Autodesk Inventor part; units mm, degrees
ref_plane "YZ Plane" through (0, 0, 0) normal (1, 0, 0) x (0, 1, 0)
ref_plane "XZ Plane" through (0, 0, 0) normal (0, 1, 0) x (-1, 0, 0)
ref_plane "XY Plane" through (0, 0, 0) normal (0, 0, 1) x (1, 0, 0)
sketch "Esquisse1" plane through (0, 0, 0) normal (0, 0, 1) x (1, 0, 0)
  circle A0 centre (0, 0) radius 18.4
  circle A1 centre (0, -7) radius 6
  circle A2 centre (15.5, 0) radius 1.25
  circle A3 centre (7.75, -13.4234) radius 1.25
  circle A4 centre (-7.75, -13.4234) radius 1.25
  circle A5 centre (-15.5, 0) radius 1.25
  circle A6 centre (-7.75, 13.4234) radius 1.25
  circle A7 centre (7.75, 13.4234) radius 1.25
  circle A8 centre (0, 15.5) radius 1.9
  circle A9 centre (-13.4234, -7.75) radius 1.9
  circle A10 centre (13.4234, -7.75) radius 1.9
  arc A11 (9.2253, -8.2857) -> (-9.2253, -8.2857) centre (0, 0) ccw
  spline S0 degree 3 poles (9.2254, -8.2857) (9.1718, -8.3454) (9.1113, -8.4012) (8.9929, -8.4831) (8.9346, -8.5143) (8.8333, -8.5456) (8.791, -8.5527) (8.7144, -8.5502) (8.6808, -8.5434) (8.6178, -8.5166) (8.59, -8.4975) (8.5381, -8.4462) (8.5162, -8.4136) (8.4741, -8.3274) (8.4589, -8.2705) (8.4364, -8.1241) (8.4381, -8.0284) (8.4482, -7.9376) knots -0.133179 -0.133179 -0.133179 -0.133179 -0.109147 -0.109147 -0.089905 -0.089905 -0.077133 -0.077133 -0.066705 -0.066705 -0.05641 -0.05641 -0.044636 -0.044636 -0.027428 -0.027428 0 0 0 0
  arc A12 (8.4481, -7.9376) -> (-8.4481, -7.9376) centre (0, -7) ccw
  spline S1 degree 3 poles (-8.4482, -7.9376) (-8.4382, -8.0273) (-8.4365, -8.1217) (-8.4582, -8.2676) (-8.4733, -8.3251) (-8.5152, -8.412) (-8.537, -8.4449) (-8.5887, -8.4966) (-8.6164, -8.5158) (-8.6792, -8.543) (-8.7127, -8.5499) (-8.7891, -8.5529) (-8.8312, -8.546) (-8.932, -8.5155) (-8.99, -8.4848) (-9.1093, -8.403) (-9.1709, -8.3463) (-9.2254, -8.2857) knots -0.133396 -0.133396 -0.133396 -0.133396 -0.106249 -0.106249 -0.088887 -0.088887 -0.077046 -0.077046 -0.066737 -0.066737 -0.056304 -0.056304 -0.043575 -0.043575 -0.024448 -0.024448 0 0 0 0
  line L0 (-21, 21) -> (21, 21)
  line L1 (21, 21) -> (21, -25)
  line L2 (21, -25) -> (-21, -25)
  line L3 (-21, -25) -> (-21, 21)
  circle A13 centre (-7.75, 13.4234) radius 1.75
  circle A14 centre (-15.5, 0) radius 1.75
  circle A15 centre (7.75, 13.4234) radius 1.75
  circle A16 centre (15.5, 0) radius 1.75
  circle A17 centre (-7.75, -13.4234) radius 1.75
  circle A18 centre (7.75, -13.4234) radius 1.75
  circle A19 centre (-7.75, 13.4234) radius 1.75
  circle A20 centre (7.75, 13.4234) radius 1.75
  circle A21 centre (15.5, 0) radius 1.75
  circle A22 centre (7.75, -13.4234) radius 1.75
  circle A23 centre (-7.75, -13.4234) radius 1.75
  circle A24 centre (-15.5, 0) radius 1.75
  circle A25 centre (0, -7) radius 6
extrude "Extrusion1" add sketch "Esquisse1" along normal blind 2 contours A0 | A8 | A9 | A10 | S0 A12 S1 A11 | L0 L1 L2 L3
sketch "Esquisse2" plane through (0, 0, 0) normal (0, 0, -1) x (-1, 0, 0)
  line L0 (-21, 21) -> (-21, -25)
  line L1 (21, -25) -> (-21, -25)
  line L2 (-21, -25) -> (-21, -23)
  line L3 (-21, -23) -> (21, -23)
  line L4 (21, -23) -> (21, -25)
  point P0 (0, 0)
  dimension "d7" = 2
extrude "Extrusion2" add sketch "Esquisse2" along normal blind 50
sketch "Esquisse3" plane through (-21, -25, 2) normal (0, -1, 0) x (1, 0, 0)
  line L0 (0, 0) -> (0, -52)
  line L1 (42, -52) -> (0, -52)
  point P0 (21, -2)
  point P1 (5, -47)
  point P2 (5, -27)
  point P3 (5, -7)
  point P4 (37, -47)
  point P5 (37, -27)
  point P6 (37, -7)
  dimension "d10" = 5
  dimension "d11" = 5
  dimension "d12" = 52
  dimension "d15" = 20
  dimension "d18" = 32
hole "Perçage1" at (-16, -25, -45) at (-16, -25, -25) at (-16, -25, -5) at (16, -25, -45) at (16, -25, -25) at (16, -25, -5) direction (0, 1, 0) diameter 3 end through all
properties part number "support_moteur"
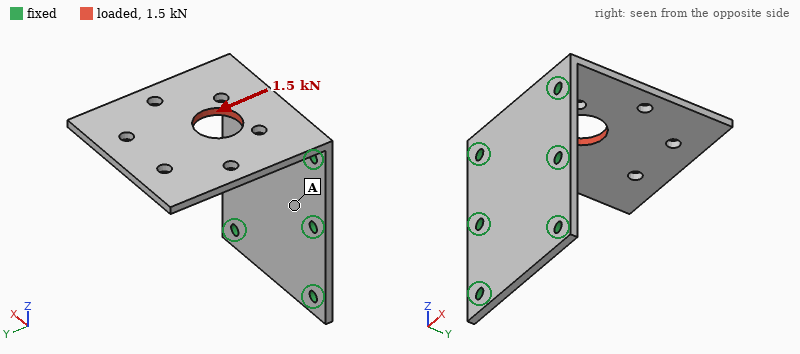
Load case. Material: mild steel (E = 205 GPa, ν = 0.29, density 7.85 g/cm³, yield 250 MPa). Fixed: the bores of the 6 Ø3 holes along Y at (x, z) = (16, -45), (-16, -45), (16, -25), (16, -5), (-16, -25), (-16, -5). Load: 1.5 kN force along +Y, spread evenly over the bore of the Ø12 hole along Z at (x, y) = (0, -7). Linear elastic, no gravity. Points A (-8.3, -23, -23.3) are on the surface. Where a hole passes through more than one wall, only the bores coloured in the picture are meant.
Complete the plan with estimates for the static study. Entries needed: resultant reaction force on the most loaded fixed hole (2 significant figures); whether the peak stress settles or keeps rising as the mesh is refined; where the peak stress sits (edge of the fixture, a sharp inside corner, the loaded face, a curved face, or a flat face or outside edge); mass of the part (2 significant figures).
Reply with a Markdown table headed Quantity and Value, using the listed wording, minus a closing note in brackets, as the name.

| Quantity | Value |
|---|---|
| resultant reaction force on the most loaded fixed hole | 810 N |
| whether the peak stress settles or keeps rising as the mesh is refined | keeps rising |
| where the peak stress sits | edge of the fixture |
| mass of the part | 60 g |
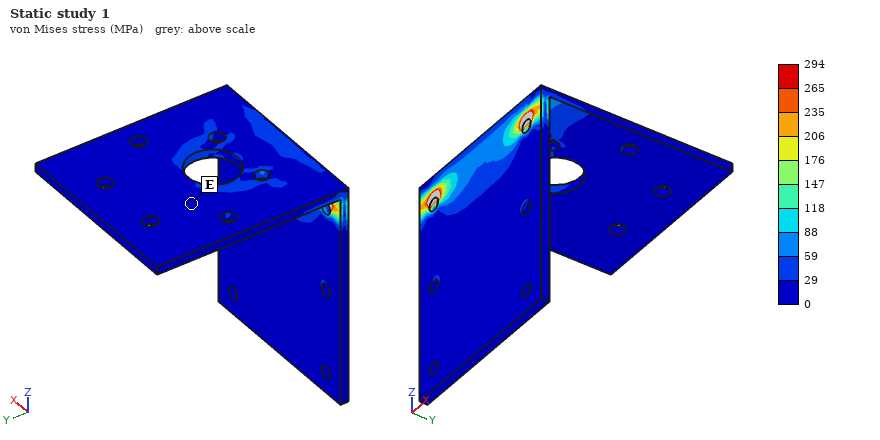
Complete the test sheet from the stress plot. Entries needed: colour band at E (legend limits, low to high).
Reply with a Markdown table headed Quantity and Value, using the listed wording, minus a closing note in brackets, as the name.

| Quantity | Value |
|---|---|
| colour band at E | 0 to 29 MPa |
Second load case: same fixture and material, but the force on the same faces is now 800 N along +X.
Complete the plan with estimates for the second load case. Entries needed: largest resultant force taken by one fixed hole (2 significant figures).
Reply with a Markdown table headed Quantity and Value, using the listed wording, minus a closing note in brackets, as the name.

| Quantity | Value |
|---|---|
| largest resultant force taken by one fixed hole | 580 N |
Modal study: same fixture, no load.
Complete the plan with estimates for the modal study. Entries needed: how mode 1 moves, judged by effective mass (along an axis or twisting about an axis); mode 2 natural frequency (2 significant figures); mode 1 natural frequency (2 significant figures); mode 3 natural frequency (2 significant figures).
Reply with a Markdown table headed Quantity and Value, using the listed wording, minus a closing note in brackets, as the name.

| Quantity | Value |
|---|---|
| how mode 1 moves, judged by effective mass | along Z |
| mode 2 natural frequency | 1800 Hz |
| mode 1 natural frequency | 650 Hz |
| mode 3 natural frequency | 4200 Hz |
